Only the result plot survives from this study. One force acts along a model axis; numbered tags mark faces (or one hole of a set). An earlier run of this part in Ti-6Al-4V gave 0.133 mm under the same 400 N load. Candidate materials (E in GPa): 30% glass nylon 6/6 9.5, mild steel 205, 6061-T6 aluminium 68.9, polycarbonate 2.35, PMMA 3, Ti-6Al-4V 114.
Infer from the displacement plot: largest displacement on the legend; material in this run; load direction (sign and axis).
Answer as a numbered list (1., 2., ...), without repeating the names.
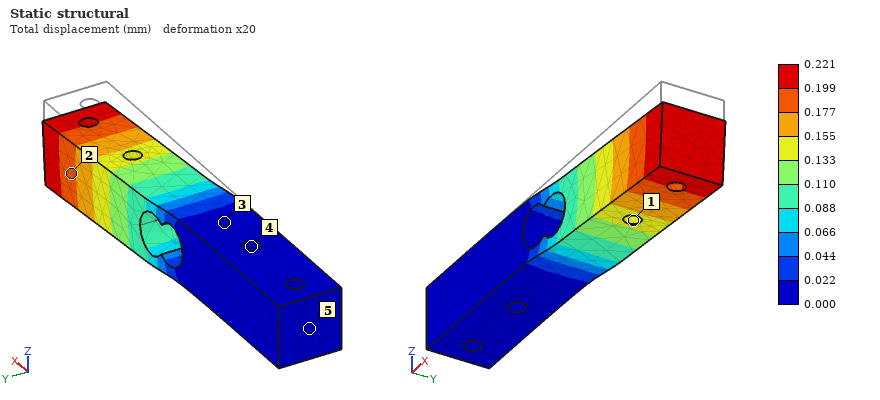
1. 0.221 mm
2. 6061-T6 aluminium
3. -Z
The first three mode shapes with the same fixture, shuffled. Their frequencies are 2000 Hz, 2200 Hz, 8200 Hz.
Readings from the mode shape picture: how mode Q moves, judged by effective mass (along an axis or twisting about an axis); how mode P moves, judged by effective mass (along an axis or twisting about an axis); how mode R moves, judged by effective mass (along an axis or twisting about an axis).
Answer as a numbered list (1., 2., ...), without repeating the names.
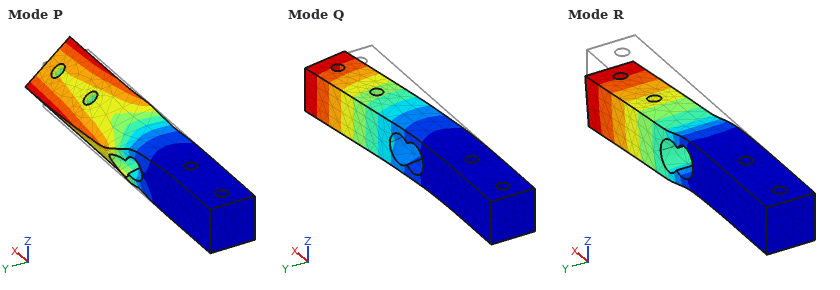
1. along Y
2. twisting about X
3. along Z
